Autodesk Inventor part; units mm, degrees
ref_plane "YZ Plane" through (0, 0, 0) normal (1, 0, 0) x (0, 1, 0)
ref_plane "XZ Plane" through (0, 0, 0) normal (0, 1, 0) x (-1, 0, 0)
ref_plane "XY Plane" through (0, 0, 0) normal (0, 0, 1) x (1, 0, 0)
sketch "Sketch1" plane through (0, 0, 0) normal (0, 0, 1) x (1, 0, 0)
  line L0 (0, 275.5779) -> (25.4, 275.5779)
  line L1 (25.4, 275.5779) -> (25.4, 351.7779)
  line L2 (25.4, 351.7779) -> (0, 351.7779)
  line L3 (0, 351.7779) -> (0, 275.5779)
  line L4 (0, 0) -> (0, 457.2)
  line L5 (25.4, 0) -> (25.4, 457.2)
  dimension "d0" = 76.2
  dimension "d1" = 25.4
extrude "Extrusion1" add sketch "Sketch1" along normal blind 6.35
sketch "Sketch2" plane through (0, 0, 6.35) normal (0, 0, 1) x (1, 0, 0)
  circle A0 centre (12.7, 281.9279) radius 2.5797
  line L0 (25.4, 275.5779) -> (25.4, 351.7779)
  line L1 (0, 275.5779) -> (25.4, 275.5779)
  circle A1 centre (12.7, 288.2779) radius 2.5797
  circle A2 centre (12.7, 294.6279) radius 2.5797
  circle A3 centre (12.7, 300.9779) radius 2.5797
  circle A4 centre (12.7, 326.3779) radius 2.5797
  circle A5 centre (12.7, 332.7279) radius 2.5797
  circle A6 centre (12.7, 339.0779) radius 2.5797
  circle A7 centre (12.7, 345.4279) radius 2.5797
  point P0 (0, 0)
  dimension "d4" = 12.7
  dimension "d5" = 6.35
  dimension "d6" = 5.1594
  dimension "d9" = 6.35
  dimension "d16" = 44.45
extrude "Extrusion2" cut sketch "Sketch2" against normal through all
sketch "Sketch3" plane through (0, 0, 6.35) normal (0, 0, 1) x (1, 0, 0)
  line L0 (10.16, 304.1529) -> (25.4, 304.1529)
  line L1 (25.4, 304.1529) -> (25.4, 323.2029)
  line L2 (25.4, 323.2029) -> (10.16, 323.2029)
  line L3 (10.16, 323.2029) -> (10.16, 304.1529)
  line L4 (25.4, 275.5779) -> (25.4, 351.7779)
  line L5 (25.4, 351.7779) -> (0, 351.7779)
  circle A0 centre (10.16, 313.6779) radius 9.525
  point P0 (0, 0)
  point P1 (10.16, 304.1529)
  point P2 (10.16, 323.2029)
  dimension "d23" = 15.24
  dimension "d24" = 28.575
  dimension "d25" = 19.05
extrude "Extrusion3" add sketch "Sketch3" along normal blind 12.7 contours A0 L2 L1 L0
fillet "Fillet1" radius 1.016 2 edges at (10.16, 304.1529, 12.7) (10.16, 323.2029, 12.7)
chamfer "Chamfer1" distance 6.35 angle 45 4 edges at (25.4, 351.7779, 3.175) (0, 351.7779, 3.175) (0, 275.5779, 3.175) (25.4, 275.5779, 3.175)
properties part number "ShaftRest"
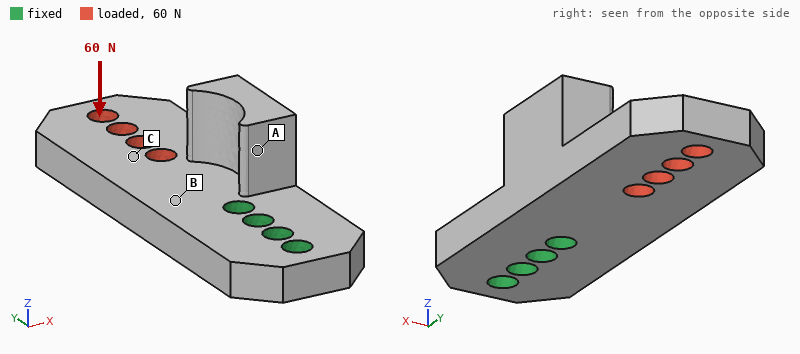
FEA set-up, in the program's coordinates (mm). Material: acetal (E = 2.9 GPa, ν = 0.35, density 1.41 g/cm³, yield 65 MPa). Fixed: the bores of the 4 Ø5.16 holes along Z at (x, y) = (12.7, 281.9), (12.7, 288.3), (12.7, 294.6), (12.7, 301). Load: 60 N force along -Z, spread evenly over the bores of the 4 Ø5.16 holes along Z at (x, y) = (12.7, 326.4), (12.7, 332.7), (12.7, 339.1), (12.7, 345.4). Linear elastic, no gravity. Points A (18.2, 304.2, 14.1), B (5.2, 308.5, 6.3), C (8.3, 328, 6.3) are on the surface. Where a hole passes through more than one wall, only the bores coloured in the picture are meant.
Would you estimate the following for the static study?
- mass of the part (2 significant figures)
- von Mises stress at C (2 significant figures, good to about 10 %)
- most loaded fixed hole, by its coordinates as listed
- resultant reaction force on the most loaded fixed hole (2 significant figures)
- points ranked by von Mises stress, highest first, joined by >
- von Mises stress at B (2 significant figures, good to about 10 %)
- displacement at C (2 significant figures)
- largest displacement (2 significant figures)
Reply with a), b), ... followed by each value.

a) 18 g
b) 3.2 MPa
c) (12.7, 301)
d) 130 N
e) B > C > A
f) 6.9 MPa
g) 0.30 mm
h) 0.76 mm
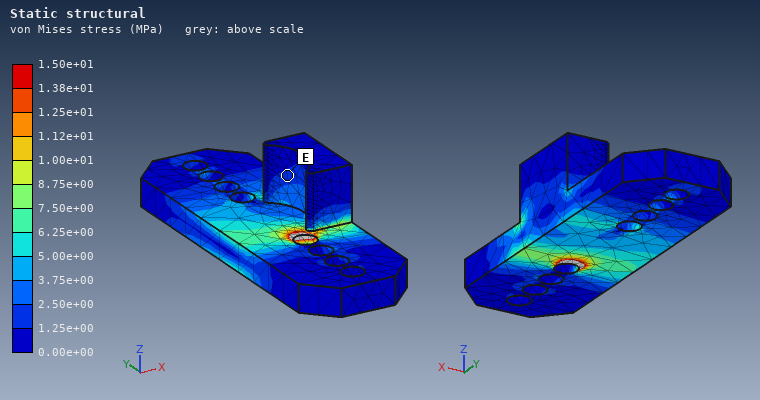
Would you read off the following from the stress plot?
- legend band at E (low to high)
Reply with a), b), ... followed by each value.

a) 1.25e+00 to 2.50e+00 MPa
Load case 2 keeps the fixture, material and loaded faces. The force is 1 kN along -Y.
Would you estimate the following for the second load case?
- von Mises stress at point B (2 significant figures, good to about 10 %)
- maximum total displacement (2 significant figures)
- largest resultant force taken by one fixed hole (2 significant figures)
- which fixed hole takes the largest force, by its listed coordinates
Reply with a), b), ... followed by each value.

a) 5.2 MPa
b) 0.13 mm
c) 680 N
d) (12.7, 301)
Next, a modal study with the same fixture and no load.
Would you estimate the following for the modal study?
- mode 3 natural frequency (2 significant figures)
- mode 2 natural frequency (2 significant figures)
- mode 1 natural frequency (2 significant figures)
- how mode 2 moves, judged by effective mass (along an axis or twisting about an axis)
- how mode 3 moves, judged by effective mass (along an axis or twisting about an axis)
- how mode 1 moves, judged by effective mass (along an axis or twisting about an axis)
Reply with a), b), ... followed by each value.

a) 1900 Hz
b) 1600 Hz
c) 690 Hz
d) along X
e) twisting about Y
f) along Z
